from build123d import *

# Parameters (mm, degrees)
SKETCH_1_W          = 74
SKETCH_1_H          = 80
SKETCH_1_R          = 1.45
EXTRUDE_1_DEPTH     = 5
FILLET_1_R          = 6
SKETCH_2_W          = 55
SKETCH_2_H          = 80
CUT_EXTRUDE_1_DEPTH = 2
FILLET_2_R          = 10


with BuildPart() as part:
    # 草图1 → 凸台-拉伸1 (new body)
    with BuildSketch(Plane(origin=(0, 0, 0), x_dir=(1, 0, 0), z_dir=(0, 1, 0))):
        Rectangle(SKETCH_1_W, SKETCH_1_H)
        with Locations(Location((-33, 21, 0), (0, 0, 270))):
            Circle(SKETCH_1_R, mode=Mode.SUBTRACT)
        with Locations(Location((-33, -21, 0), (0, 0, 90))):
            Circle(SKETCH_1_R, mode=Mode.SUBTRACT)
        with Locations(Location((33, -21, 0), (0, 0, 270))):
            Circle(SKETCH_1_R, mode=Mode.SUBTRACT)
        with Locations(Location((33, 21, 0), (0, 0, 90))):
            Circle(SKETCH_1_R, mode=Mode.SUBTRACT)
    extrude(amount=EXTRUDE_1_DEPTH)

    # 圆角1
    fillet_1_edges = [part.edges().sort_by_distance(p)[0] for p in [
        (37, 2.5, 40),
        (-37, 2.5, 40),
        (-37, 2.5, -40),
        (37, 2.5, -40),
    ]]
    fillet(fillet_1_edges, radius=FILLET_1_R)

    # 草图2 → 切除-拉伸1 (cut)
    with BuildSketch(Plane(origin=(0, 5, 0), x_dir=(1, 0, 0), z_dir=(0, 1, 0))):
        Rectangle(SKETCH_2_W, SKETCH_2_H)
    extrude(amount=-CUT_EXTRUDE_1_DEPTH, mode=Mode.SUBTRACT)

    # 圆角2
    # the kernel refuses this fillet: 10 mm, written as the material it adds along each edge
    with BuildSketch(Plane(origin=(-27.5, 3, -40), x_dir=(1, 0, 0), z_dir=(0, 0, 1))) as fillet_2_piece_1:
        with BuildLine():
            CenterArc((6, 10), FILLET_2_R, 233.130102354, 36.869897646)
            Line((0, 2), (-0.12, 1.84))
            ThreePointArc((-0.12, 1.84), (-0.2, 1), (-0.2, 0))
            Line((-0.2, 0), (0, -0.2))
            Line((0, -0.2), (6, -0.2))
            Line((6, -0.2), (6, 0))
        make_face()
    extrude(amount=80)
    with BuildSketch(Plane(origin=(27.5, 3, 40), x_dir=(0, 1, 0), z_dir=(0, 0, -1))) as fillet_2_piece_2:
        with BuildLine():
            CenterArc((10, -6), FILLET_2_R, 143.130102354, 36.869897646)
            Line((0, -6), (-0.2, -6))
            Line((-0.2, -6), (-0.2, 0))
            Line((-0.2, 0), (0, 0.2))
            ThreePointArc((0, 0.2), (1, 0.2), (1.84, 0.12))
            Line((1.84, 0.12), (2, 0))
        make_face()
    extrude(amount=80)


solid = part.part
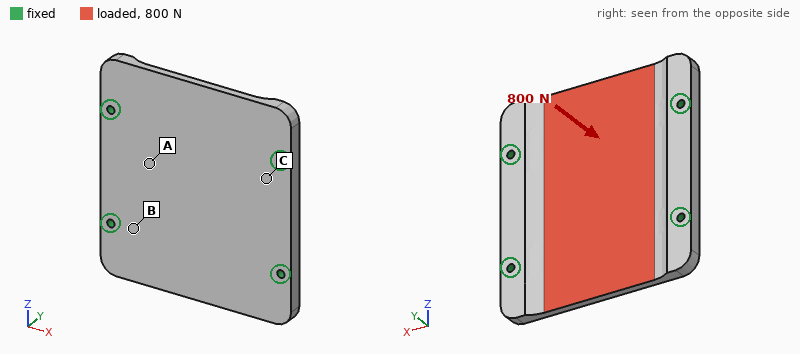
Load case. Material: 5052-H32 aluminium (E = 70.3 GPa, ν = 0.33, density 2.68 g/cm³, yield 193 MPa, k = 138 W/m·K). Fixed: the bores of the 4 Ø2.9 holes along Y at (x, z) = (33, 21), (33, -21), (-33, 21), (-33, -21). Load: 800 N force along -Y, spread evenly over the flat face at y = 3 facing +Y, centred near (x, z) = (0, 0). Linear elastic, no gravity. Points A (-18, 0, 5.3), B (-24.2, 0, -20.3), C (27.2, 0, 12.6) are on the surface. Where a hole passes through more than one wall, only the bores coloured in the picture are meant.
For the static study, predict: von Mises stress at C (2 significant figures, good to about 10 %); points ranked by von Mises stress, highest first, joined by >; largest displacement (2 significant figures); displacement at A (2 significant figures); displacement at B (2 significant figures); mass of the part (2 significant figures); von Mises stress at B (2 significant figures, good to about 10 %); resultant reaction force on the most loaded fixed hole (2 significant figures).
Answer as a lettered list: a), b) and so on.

a) 11 MPa
b) B > C > A
c) 59 µm
d) 25 µm
e) 9.6 µm
f) 57 g
g) 20 MPa
h) 310 N
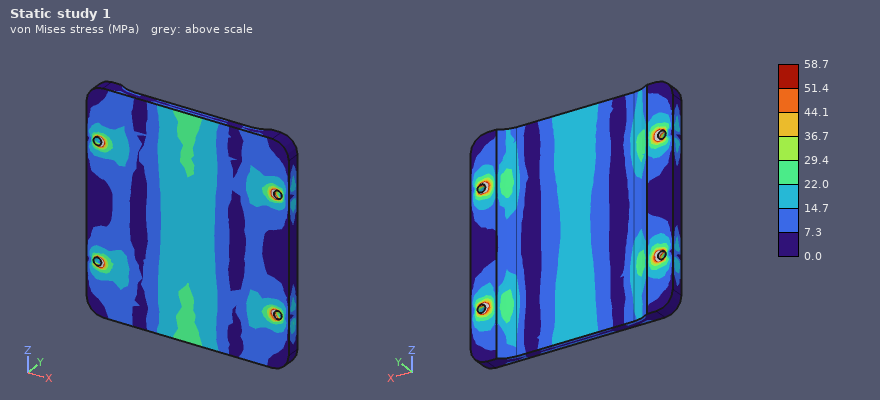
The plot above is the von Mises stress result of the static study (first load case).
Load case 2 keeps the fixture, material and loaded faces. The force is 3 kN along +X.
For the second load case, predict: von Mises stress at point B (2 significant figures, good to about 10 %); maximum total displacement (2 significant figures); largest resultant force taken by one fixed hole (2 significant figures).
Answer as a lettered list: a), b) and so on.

a) 11 MPa
b) 6.6 µm
c) 750 N
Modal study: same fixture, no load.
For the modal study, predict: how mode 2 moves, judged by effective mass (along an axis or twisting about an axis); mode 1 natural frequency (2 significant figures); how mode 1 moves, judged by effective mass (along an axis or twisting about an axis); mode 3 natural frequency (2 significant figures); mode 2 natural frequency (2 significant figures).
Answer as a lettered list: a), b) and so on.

a) twisting about X
b) 4100 Hz
c) along Y
d) 5500 Hz
e) 4500 Hz
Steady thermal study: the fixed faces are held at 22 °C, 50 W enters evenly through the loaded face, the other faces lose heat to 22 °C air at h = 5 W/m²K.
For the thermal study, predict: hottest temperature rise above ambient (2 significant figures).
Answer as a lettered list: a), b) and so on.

a) 20 K
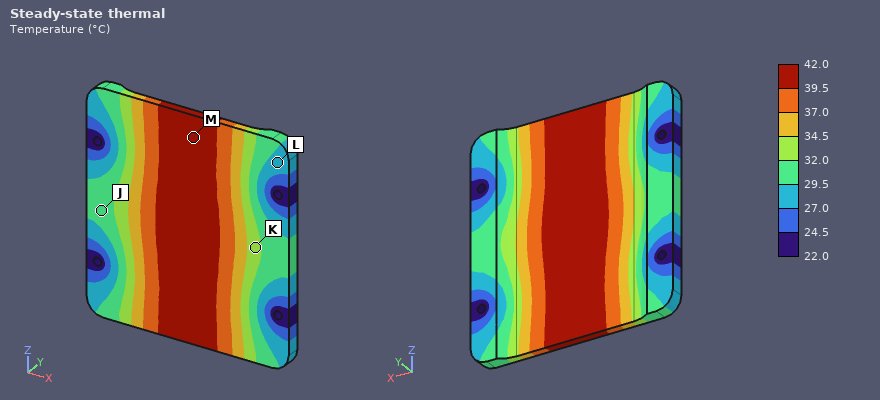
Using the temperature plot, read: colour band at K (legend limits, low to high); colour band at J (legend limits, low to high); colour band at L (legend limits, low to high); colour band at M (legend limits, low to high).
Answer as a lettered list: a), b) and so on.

a) 32.0 to 34.5 °C
b) 29.5 to 32.0 °C
c) 27.0 to 29.5 °C
d) 39.5 to 42.0 °C
